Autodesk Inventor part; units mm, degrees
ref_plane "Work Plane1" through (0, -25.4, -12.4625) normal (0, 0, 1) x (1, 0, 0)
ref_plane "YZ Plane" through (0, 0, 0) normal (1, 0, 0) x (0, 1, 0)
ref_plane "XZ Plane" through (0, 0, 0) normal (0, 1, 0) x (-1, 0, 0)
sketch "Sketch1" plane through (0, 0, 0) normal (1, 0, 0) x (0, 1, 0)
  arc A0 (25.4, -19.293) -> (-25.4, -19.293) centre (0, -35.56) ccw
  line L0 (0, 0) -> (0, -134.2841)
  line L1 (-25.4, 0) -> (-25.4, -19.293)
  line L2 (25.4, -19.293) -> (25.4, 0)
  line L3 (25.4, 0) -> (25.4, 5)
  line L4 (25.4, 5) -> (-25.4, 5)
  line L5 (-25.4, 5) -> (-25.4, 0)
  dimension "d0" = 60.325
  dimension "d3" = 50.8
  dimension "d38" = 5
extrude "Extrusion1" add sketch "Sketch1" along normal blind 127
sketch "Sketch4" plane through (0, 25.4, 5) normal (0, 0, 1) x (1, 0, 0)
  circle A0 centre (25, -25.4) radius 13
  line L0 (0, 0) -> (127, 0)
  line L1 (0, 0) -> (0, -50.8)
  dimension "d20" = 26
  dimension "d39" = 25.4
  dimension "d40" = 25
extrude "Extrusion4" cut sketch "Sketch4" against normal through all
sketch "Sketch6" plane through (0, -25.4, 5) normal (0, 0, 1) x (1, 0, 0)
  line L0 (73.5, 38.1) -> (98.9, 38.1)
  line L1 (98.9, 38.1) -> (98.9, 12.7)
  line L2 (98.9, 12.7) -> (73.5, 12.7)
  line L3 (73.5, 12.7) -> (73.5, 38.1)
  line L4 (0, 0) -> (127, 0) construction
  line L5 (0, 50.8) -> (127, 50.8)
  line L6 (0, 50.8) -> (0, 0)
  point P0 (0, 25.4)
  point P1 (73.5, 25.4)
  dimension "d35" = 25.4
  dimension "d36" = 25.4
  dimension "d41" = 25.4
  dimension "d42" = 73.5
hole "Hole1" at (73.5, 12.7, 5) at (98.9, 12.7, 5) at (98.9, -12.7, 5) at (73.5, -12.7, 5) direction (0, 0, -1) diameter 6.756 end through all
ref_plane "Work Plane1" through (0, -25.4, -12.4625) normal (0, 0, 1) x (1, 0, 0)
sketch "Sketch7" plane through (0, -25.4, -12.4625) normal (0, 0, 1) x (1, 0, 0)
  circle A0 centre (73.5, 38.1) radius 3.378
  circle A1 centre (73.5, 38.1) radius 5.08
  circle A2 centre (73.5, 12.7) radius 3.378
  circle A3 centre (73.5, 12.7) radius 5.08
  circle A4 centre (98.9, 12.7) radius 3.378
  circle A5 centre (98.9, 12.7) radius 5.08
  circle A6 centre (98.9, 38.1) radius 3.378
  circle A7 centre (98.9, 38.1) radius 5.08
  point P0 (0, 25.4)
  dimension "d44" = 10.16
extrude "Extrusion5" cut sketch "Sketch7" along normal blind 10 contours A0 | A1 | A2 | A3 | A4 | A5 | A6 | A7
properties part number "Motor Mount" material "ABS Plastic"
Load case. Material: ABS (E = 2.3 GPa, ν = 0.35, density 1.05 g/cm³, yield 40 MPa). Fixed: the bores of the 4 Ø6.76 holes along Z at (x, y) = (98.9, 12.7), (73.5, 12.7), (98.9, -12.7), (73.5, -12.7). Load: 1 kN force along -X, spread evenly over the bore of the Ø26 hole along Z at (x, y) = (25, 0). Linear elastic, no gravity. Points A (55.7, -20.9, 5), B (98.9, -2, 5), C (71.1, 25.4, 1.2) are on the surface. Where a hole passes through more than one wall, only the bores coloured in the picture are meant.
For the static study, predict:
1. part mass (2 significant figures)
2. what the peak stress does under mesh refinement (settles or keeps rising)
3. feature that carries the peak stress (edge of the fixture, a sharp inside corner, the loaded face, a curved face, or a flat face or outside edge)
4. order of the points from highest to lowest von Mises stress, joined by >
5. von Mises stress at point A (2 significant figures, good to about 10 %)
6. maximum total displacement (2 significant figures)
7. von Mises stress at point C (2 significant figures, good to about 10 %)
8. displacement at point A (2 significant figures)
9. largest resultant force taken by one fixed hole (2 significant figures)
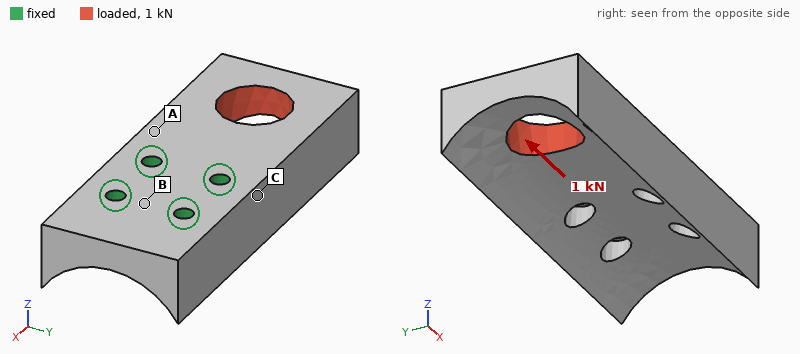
89 g
keeps rising
edge of the fixture
A > C > B
2.3 MPa
0.11 mm
1.2 MPa
0.020 mm
400 N
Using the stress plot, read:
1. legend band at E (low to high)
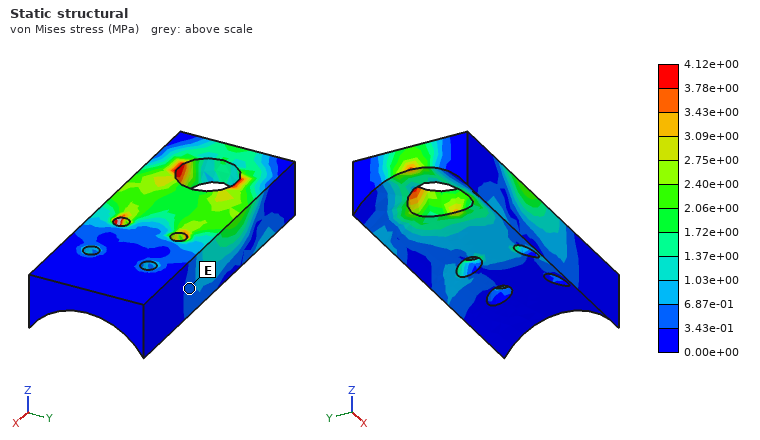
3.43e-01 to 6.87e-01 MPa
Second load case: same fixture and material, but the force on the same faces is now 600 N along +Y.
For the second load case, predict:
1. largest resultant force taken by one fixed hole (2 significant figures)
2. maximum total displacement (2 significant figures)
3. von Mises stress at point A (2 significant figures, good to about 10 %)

730 N
0.33 mm
2.8 MPa
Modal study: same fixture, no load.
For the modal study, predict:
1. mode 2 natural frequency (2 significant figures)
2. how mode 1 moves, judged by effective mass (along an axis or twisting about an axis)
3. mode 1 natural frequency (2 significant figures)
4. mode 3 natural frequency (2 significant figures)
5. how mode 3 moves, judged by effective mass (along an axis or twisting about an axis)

1200 Hz
along Z
660 Hz
1500 Hz
along Y
